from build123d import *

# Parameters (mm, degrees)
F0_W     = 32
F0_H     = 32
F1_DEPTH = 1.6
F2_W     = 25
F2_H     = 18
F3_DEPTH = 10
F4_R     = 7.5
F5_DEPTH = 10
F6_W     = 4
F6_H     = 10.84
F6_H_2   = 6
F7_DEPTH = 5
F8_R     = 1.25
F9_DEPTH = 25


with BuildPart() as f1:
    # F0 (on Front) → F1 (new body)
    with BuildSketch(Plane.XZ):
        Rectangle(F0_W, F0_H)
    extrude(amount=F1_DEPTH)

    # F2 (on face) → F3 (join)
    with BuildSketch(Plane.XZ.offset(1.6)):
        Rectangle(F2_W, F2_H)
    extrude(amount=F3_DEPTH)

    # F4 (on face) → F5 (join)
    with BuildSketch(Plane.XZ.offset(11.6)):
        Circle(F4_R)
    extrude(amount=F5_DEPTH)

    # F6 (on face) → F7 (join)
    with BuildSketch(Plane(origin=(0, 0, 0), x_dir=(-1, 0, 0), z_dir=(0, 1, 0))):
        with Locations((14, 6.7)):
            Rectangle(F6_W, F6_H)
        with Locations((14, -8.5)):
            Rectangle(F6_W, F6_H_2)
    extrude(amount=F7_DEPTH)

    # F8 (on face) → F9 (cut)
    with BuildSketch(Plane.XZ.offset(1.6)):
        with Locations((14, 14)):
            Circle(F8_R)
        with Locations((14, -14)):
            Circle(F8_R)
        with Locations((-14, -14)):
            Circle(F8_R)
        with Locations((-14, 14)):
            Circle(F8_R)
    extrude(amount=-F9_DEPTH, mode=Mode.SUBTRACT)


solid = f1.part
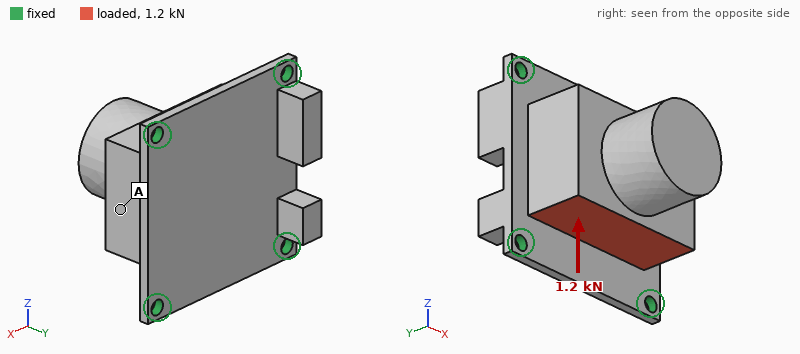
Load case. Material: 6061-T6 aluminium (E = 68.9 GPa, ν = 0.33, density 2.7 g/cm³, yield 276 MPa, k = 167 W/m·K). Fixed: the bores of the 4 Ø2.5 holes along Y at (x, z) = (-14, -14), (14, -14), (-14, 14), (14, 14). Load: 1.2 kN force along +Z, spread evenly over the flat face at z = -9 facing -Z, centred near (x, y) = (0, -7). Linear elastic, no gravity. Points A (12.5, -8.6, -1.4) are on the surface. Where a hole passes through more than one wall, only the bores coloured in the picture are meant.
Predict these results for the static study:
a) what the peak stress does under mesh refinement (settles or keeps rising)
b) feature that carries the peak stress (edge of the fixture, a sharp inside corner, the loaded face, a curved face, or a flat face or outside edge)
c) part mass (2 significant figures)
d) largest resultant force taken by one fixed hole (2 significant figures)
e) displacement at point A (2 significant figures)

keeps rising
edge of the fixture
22 g
390 N
14 µm
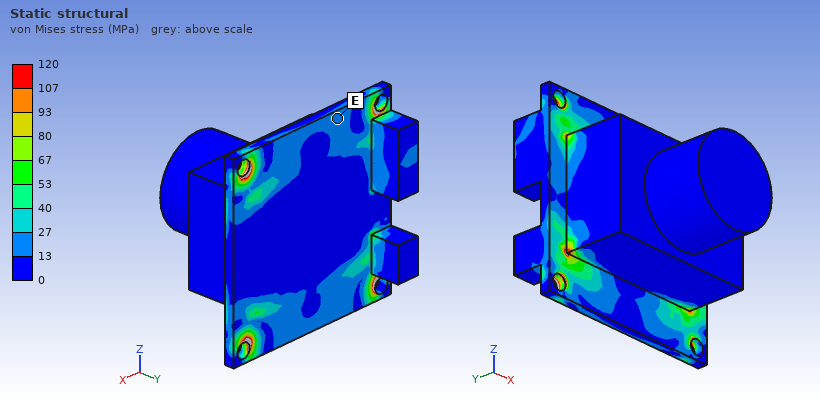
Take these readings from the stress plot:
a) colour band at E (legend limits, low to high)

13 to 27 MPa
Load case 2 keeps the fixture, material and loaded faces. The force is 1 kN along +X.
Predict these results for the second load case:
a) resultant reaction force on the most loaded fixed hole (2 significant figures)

350 N
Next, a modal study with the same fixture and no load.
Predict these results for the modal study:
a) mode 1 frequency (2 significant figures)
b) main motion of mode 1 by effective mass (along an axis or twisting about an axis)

6400 Hz
along Y
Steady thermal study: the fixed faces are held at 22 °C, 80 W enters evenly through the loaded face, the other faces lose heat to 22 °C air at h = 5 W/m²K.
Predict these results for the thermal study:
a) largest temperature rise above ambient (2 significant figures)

70 K
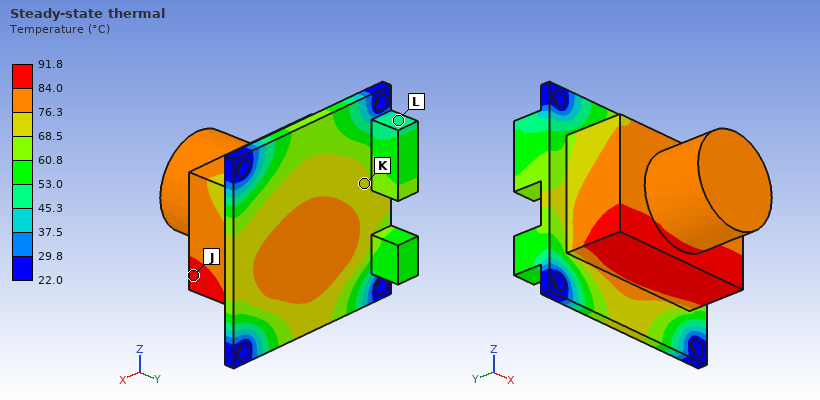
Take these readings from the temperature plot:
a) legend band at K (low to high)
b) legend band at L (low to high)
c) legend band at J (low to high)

68.5 to 76.3 °C
45.3 to 53.0 °C
84.0 to 91.8 °C
